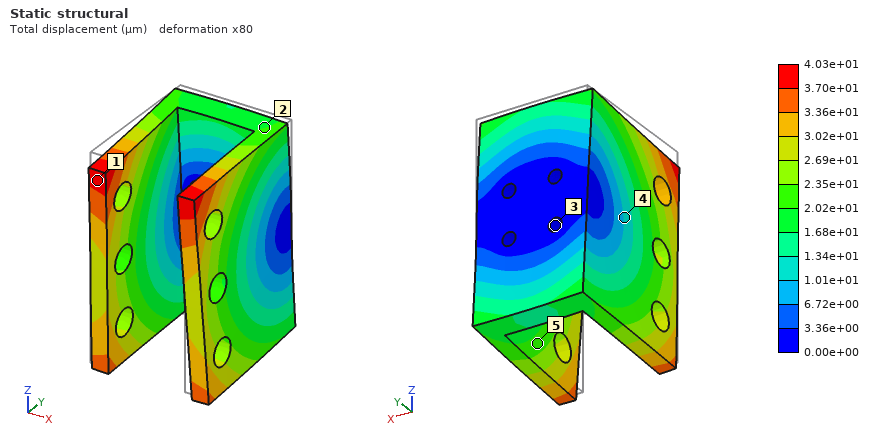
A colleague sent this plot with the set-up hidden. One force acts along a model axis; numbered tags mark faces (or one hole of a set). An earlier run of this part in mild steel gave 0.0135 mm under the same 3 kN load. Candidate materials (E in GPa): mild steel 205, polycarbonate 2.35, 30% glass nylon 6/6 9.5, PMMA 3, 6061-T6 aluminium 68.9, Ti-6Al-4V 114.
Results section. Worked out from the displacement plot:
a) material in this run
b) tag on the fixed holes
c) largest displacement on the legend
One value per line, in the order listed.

6061-T6 aluminium
3
4.03e+01 µm
